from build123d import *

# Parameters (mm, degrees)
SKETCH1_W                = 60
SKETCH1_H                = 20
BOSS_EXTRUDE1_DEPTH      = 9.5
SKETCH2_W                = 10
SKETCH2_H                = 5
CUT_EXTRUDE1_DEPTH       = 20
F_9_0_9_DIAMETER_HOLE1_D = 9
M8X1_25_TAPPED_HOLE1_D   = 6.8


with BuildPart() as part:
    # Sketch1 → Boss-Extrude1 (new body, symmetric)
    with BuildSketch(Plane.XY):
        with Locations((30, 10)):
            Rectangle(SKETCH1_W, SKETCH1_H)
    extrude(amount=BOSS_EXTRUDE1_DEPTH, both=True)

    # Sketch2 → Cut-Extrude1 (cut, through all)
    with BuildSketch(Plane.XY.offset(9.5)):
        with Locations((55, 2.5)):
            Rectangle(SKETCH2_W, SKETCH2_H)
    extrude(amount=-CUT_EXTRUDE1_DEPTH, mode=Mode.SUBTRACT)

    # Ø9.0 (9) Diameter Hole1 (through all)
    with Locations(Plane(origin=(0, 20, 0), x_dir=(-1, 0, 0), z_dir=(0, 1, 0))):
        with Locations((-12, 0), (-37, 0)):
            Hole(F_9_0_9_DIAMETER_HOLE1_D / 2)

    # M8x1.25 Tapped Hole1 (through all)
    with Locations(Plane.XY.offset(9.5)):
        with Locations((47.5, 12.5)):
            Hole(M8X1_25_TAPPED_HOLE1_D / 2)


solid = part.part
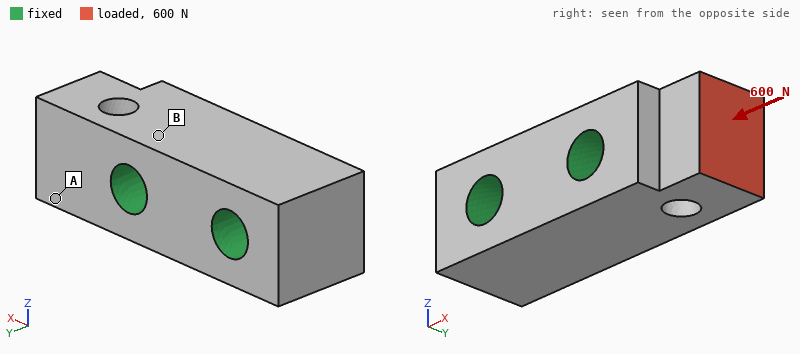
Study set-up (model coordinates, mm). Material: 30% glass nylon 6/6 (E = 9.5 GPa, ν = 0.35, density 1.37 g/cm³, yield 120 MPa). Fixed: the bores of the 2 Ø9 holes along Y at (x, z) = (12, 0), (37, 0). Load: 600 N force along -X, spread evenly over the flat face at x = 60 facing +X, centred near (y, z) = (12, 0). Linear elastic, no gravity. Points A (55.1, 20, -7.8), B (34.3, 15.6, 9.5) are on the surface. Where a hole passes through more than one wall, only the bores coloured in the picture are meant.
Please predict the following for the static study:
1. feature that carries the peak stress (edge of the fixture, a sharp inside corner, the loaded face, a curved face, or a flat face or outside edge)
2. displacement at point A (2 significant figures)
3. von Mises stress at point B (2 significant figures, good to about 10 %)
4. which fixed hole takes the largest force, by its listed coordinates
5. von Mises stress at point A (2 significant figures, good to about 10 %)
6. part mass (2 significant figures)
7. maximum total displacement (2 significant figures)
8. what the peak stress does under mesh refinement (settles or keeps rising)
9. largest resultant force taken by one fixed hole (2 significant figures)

edge of the fixture
6.5 µm
0.87 MPa
(37, 0)
2.7 MPa
26 g
7.8 µm
keeps rising
570 N
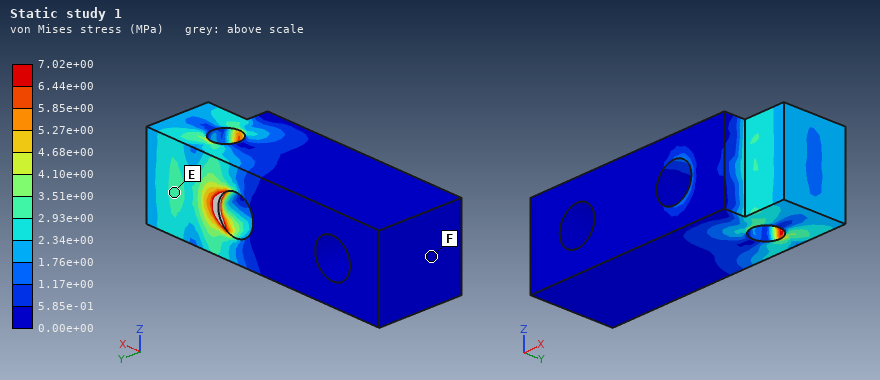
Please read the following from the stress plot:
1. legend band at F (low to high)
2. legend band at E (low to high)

0.00e+00 to 5.85e-01 MPa
2.93e+00 to 3.51e+00 MPa
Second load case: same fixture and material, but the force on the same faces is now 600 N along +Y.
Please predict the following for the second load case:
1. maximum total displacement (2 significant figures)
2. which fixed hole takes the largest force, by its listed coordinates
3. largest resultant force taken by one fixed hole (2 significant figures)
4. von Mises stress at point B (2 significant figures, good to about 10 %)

42 µm
(37, 0)
630 N
1.9 MPa
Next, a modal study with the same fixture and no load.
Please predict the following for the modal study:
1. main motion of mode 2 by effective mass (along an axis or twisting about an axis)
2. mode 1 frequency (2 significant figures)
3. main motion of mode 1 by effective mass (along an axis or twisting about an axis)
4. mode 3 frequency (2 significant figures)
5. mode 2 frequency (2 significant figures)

along Y
11 kHz
along Z
18 kHz
13 kHz
